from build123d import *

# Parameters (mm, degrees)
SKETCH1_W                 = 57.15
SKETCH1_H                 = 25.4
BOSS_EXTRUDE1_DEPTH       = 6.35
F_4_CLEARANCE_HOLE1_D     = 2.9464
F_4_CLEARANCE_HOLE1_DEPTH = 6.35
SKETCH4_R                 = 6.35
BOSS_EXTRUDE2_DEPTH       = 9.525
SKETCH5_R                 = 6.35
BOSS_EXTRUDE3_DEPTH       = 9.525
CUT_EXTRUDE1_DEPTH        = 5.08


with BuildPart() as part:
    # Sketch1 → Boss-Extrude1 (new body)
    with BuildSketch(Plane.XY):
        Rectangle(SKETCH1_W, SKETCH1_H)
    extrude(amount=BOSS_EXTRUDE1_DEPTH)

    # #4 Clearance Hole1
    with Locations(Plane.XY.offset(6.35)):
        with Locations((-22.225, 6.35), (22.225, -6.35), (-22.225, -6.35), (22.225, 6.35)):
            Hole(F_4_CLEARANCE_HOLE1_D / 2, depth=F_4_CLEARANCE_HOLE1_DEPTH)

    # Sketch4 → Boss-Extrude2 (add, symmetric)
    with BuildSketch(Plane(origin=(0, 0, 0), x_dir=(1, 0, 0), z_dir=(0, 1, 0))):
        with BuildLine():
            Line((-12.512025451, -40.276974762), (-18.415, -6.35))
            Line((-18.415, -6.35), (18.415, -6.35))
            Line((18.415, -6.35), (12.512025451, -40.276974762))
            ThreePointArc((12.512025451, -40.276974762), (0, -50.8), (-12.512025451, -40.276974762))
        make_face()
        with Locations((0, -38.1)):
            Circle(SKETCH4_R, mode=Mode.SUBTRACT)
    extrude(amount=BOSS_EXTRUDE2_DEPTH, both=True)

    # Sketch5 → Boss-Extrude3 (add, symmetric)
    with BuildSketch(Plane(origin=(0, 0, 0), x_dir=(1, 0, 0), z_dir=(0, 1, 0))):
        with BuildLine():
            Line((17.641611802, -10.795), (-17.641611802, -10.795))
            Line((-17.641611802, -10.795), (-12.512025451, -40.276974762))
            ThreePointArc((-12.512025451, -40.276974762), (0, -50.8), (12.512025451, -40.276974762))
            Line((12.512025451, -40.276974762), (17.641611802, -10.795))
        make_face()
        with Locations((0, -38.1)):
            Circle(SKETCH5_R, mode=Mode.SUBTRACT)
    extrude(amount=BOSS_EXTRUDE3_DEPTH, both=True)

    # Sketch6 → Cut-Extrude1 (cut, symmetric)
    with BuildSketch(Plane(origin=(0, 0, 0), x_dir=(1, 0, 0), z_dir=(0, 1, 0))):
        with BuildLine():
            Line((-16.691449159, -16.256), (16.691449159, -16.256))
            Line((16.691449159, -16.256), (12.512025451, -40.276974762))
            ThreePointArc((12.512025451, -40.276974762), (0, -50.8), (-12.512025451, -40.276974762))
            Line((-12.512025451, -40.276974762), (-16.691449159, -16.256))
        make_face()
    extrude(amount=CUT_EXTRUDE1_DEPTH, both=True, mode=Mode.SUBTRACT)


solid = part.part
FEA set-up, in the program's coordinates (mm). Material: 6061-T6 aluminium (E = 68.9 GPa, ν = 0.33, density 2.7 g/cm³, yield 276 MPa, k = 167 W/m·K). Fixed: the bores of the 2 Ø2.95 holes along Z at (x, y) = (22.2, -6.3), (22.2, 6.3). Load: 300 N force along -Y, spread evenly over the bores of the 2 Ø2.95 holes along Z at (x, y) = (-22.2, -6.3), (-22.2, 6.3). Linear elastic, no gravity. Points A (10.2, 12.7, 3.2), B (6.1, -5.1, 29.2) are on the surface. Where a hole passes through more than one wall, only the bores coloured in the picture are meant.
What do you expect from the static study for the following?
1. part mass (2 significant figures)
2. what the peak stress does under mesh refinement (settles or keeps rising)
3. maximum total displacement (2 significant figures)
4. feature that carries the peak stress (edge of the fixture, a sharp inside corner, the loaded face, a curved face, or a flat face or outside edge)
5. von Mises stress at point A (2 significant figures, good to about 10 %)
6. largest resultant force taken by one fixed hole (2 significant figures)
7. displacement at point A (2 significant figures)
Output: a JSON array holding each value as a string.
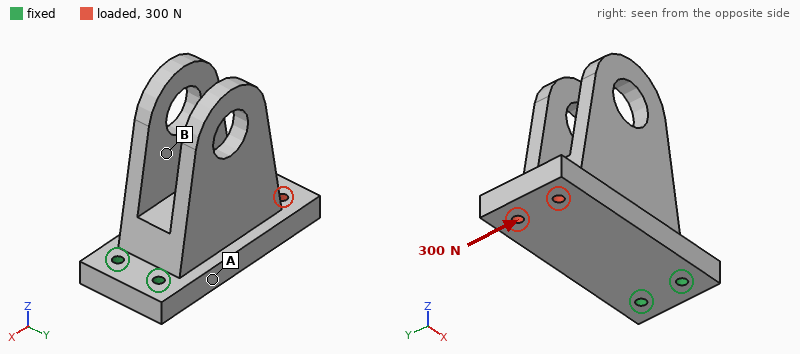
["61 g", "keeps rising", "24 µm", "edge of the fixture", "11 MPa", "930 N", "5.5 µm"]
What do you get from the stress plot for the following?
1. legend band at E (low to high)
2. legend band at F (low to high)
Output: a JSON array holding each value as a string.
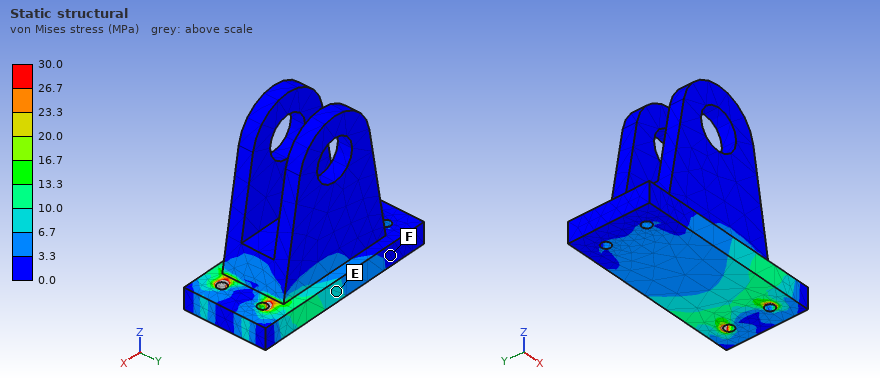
["6.7 to 10.0 MPa", "0.0 to 3.3 MPa"]
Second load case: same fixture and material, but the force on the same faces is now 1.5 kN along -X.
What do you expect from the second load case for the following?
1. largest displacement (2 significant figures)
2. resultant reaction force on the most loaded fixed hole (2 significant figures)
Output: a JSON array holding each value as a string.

["13 µm", "760 N"]
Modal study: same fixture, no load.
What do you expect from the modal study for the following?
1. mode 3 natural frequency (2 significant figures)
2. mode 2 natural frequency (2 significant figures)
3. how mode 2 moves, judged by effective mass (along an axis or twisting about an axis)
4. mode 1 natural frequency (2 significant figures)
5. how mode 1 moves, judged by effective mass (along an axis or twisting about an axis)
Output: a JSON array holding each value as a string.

["3700 Hz", "2800 Hz", "along Y", "1500 Hz", "along Z"]
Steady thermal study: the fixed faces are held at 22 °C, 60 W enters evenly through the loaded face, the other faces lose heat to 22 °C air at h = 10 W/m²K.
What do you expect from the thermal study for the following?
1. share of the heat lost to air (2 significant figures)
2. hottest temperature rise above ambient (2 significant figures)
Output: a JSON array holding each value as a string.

["4.5 %", "67 K"]
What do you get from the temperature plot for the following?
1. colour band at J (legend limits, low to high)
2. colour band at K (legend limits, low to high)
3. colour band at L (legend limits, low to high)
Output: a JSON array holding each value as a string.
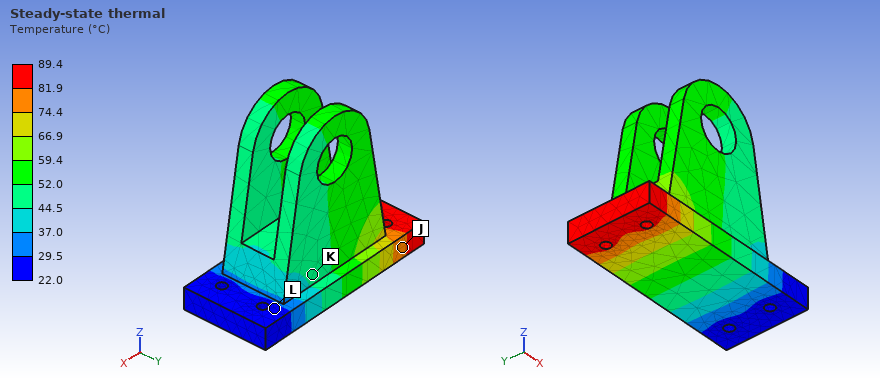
["74.4 to 81.9 °C", "44.5 to 52.0 °C", "22.0 to 29.5 °C"]
